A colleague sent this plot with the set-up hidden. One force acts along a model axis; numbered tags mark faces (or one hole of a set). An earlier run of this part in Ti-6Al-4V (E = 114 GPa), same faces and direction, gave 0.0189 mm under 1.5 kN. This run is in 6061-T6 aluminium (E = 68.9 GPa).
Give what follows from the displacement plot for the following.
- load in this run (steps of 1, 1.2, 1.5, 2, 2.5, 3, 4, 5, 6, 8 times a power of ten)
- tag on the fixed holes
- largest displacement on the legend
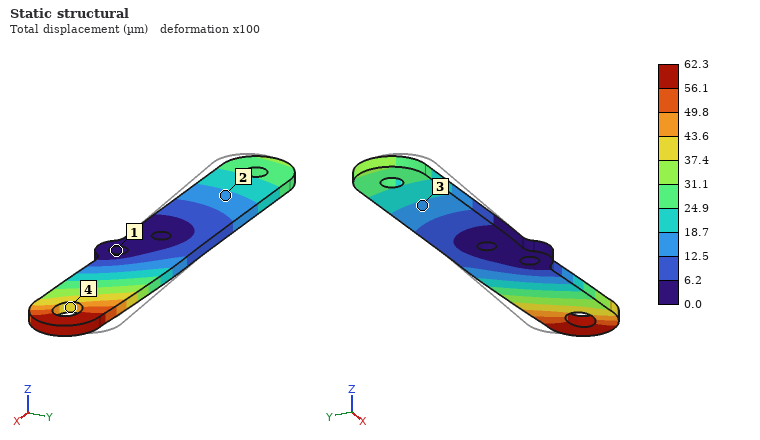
3 kN
1
62.3 µm
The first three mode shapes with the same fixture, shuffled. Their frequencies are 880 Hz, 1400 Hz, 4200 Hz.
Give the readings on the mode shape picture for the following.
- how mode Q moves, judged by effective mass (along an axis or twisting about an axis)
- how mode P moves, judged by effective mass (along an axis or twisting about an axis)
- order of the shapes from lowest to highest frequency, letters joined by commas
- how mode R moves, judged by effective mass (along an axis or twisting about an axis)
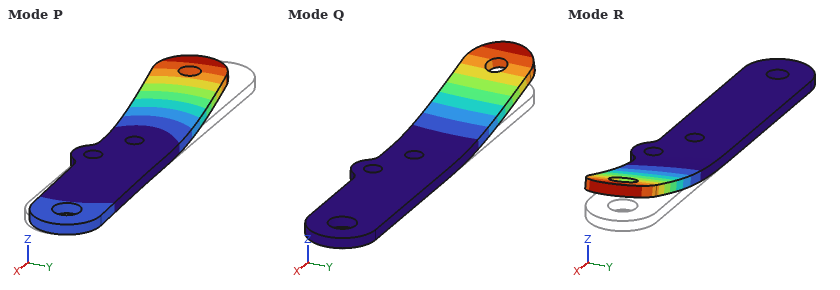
along Z
along Y
Q, R, P
along Z
